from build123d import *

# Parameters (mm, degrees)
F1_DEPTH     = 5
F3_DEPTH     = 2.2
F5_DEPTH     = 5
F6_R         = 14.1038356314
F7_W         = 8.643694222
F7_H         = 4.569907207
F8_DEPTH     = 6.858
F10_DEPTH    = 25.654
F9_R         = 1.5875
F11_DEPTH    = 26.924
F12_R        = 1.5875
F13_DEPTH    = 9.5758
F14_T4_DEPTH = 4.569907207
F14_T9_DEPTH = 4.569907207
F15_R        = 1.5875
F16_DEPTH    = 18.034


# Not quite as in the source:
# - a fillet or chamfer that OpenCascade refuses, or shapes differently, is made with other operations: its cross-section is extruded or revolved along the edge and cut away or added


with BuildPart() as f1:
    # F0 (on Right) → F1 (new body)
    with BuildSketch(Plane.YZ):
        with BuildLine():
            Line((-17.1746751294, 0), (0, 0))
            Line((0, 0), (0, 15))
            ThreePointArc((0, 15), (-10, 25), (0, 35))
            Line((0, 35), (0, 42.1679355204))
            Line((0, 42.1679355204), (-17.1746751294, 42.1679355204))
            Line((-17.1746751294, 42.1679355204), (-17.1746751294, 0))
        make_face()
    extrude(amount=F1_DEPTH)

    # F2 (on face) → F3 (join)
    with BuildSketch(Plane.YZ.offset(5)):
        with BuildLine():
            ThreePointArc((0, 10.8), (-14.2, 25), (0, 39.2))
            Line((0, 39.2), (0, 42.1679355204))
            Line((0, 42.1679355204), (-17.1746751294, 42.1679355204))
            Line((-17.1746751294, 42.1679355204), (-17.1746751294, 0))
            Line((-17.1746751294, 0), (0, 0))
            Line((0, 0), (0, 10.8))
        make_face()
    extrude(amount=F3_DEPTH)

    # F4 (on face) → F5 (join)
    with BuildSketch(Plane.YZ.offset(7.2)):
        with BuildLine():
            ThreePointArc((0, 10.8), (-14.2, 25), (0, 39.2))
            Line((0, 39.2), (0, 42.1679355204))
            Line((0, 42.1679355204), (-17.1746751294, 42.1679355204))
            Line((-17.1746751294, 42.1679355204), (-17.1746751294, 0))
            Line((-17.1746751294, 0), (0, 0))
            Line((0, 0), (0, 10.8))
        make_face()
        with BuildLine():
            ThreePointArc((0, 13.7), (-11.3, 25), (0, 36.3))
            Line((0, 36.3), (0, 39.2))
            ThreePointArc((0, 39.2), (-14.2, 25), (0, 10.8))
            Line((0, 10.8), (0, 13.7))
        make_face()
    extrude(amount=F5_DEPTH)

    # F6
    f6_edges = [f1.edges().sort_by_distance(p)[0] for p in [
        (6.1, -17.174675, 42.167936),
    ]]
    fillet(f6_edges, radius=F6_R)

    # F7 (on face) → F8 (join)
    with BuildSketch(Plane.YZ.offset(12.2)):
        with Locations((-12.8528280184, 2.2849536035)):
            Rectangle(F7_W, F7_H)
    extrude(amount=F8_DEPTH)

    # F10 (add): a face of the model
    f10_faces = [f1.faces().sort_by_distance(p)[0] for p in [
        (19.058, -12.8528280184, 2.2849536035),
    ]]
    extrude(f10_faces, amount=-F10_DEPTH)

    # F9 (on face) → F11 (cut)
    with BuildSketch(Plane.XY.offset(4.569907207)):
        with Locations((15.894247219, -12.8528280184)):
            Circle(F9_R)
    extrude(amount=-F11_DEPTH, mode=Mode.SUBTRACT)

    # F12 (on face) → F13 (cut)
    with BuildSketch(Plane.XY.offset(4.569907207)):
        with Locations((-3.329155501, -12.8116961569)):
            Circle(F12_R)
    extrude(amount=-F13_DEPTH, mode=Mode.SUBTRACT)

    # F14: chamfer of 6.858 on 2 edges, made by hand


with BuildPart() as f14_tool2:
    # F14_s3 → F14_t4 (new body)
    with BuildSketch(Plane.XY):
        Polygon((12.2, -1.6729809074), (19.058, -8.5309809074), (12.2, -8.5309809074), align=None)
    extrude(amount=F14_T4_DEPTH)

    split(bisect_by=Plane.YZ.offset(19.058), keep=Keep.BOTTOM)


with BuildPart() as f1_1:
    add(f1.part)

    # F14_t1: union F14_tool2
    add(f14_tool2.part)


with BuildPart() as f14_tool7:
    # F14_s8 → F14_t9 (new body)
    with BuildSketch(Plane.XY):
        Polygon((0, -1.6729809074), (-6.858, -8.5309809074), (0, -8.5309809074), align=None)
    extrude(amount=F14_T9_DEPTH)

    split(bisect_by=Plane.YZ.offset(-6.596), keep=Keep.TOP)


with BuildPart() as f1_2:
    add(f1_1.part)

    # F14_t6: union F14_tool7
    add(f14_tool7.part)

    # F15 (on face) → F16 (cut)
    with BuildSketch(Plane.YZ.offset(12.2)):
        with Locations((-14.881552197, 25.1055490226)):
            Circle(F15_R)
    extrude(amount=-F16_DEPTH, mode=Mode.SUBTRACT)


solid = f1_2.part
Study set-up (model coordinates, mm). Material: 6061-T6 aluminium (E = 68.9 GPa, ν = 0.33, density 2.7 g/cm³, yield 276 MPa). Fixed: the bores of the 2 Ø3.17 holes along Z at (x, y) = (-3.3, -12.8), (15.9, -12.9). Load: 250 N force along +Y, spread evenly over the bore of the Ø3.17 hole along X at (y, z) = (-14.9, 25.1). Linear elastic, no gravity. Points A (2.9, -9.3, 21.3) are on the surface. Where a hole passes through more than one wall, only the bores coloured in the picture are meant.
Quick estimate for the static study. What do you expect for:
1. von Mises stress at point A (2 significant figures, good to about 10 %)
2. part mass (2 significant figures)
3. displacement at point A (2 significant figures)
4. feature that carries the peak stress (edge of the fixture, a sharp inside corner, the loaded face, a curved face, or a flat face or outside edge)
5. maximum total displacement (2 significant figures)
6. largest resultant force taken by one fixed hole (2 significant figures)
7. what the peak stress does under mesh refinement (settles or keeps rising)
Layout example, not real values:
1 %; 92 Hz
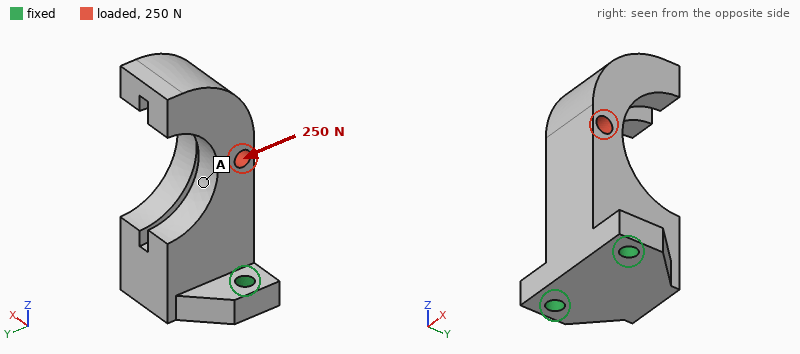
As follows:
18 MPa; 17 g; 35 µm; edge of the fixture; 87 µm; 140 N; keeps rising
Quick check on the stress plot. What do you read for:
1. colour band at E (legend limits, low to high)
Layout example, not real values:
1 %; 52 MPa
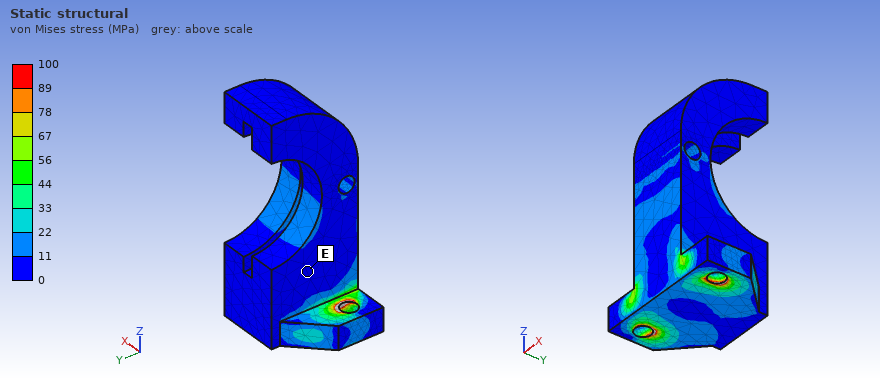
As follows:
0 to 11 MPa
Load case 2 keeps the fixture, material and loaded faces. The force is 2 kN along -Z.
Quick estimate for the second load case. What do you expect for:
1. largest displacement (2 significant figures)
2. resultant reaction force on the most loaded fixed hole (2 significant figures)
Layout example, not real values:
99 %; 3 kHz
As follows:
0.11 mm; 1.1 kN
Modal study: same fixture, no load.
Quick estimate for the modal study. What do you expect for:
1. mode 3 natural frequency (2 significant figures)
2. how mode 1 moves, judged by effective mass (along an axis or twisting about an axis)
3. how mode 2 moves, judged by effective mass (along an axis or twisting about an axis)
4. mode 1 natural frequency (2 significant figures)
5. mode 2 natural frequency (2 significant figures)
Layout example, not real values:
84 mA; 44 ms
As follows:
11 kHz; along Y; along X; 3100 Hz; 4500 Hz
